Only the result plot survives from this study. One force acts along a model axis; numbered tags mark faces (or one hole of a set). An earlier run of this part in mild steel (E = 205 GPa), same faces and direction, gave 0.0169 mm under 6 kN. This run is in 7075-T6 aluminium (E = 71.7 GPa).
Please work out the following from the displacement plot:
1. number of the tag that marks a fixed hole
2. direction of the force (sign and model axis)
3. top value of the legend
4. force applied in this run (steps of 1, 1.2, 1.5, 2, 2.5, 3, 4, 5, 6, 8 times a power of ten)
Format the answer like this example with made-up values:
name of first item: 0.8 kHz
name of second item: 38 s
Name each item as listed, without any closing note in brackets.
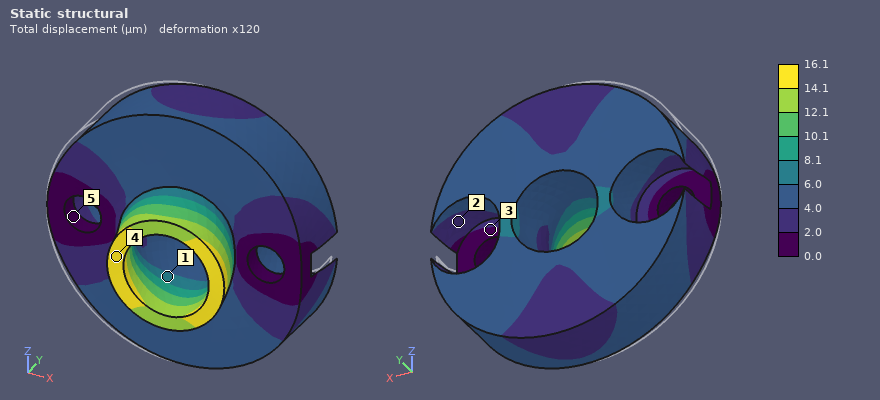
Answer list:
number of the tag that marks a fixed hole: 5
direction of the force: +X
top value of the legend: 16.1 µm
force applied in this run: 2 kN
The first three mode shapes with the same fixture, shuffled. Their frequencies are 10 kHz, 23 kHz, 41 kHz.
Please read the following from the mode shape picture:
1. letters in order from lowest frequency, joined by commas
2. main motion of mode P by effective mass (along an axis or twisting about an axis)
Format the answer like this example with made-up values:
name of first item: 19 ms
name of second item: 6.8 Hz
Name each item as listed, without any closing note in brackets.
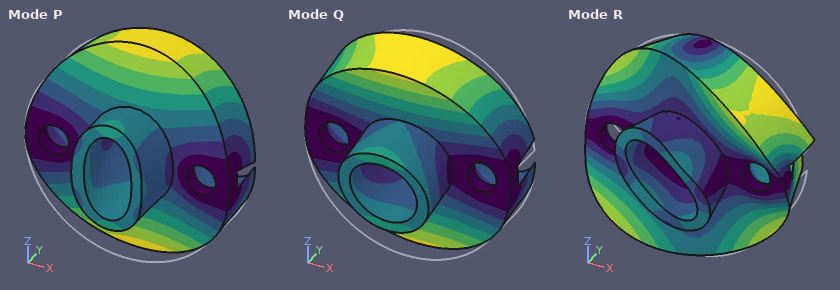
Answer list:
letters in order from lowest frequency, joined by commas: Q, P, R
main motion of mode P by effective mass: along Y
